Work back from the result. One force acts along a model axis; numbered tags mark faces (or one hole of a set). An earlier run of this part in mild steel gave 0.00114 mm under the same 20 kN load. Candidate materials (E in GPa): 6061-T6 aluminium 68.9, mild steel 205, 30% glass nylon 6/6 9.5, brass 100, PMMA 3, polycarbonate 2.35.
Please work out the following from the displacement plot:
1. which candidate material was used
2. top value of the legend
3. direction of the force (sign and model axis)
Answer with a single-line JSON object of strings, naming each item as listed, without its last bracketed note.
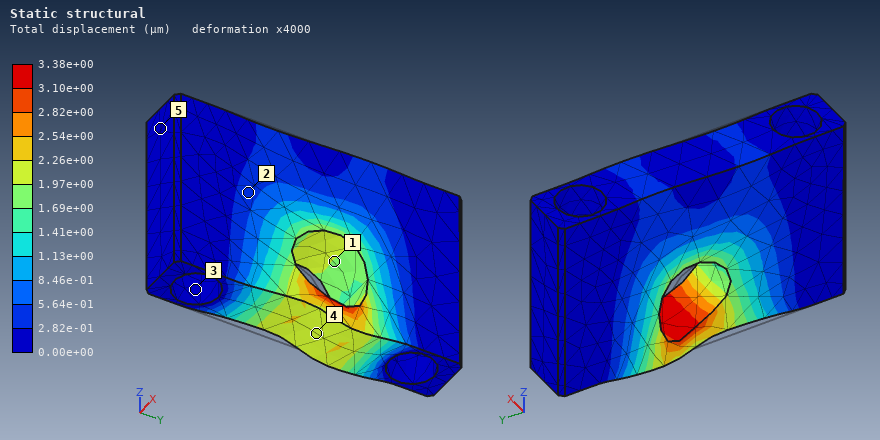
{"which candidate material was used": "6061-T6 aluminium", "top value of the legend": "3.38e+00 µm", "direction of the force": "+Y"}
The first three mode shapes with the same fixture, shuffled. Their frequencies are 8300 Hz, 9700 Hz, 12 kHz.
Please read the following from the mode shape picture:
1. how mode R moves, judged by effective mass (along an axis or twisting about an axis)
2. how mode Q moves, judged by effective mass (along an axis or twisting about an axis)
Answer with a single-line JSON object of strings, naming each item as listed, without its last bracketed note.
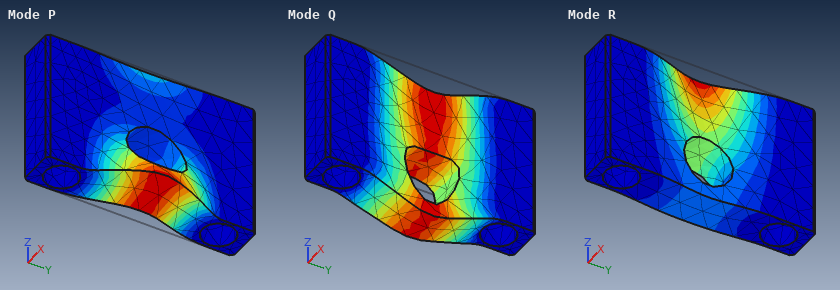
{"how mode R moves, judged by effective mass": "along X", "how mode Q moves, judged by effective mass": "along Z"}
